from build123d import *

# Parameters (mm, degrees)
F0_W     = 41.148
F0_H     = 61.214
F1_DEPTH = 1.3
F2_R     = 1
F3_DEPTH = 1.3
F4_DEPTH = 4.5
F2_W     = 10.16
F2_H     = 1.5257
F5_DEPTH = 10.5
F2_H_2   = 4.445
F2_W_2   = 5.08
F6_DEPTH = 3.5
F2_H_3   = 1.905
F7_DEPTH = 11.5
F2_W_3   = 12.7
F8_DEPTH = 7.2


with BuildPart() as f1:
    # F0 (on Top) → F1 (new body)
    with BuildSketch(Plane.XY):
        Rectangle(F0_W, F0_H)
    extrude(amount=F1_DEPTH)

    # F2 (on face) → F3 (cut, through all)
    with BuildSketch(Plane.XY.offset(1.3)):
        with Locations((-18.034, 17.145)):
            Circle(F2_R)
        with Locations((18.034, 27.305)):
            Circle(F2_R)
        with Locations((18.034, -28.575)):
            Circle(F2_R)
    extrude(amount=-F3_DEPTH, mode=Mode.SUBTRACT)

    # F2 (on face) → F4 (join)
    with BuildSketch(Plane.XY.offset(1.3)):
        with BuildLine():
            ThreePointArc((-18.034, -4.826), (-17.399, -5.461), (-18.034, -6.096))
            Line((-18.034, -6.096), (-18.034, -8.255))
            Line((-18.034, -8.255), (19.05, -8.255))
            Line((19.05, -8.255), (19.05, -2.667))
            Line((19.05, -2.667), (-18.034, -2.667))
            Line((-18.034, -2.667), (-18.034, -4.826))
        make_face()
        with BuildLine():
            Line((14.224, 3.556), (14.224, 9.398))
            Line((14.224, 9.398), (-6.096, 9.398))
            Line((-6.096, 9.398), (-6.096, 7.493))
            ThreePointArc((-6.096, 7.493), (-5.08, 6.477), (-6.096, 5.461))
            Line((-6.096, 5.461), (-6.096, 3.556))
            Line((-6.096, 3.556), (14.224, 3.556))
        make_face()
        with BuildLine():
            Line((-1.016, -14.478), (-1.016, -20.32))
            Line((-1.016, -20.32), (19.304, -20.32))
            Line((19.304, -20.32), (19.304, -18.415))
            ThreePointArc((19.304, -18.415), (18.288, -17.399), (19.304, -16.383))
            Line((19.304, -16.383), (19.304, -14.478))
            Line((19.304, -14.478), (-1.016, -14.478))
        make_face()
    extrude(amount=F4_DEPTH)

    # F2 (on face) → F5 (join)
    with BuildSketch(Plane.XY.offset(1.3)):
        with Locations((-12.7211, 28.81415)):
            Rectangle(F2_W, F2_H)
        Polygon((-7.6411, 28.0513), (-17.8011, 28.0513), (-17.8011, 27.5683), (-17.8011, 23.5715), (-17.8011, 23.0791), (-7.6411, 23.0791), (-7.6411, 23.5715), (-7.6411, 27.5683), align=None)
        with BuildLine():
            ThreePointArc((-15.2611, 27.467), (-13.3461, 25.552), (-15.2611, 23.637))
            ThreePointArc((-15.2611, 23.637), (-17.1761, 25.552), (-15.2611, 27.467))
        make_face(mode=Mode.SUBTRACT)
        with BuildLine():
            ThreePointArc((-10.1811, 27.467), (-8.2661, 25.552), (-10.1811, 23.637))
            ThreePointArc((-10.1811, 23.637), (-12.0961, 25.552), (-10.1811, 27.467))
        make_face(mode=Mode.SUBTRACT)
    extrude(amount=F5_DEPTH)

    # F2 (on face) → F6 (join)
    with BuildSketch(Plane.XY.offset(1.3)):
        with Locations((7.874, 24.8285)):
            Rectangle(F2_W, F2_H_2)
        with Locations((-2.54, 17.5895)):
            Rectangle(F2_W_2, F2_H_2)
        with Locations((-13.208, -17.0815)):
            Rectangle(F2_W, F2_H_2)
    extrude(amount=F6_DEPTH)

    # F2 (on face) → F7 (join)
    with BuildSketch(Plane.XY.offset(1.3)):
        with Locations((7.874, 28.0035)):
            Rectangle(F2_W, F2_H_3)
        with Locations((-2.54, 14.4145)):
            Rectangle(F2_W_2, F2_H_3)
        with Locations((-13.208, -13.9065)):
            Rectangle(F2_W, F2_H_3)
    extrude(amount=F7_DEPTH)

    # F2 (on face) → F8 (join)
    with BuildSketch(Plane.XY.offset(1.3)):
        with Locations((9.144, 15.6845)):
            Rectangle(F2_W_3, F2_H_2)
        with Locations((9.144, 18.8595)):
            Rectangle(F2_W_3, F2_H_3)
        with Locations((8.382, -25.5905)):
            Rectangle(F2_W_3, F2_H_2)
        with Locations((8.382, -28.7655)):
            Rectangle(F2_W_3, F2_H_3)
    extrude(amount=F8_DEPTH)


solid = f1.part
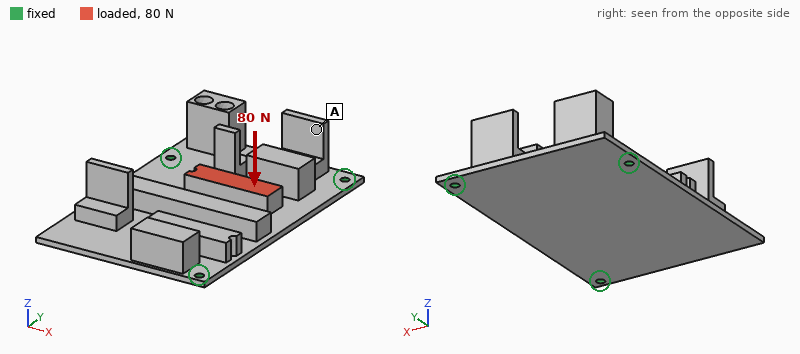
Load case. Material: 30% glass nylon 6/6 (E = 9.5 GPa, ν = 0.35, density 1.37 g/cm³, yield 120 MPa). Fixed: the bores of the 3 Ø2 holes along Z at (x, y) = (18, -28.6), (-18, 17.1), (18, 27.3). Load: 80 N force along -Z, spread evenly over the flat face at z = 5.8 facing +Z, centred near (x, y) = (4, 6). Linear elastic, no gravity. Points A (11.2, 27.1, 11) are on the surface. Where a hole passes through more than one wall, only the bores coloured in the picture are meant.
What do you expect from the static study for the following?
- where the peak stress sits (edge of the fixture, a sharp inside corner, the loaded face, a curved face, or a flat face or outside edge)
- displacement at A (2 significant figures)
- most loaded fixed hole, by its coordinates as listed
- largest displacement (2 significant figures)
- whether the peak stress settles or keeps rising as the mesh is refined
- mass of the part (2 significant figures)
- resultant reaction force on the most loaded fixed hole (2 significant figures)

edge of the fixture
0.28 mm
(-18, 17.1)
0.75 mm
keeps rising
11 g
39 N
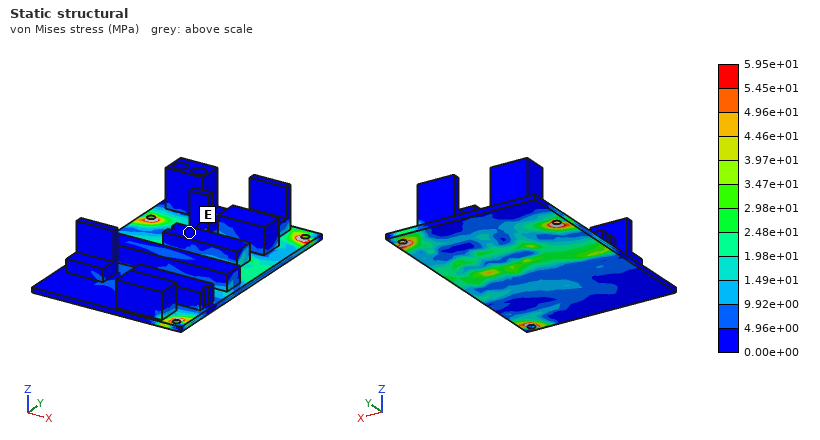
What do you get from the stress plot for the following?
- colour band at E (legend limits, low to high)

0.00e+00 to 4.96e+00 MPa
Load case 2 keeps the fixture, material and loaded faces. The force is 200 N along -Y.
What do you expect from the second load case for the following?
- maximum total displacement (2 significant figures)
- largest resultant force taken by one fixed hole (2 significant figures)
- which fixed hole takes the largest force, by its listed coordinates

0.43 mm
91 N
(18, 27.3)
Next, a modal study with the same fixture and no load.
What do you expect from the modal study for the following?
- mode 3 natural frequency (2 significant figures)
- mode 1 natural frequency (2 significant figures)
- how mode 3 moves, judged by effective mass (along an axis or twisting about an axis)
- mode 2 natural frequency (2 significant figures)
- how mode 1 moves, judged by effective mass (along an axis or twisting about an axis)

1600 Hz
650 Hz
along Z
940 Hz
along Z
